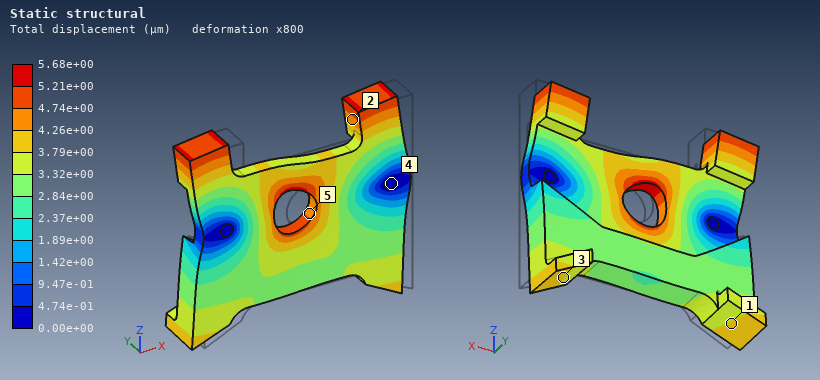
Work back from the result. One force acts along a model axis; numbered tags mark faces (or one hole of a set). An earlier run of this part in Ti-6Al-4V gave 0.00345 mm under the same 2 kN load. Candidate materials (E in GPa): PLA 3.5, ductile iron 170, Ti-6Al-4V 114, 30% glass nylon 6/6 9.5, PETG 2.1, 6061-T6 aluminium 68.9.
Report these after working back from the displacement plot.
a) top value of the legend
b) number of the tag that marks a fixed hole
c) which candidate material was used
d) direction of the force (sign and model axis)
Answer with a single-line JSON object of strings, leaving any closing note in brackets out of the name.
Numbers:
{"top value of the legend": "5.68e+00 µm", "number of the tag that marks a fixed hole": "4", "which candidate material was used": "6061-T6 aluminium", "direction of the force": "-X"}
